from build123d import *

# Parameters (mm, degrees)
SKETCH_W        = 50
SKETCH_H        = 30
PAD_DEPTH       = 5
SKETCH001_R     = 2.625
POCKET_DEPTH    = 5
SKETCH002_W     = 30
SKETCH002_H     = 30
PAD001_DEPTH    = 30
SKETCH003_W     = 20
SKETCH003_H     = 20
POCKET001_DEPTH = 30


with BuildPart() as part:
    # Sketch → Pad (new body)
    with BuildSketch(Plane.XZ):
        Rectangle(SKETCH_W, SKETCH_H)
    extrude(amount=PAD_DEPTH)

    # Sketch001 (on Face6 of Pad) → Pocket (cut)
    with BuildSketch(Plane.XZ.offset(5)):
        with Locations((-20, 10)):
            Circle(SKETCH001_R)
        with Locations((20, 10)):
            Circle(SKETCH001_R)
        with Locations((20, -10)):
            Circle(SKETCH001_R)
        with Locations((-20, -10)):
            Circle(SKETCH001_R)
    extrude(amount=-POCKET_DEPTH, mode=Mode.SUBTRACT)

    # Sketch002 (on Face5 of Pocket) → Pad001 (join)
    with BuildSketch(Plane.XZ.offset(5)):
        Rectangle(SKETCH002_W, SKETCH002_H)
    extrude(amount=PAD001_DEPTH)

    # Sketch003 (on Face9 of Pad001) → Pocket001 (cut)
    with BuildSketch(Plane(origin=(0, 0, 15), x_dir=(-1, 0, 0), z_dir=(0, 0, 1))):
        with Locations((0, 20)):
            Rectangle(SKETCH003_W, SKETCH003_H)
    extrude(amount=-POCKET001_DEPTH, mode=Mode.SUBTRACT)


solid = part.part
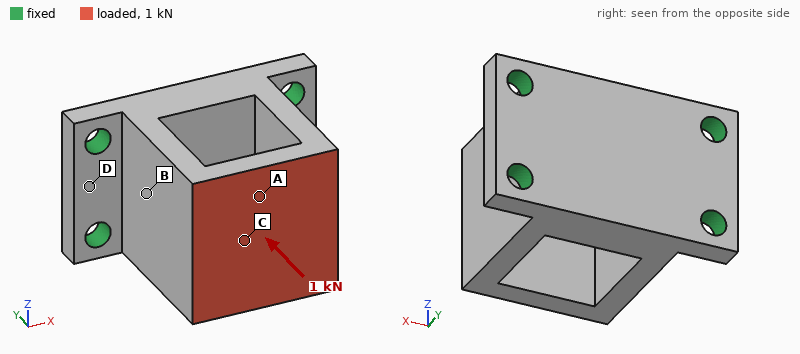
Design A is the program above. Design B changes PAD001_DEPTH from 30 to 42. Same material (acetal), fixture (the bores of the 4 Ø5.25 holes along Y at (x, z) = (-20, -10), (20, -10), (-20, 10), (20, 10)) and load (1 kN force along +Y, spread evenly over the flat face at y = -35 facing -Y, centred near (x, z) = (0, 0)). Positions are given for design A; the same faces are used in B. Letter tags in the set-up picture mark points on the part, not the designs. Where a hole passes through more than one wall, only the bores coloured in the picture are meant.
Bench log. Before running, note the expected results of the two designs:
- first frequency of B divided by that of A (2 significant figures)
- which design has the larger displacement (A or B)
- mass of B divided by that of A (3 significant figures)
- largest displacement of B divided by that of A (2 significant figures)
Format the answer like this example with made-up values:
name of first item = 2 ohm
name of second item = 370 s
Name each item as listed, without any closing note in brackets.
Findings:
first frequency of B divided by that of A = 0.64
which design has the larger displacement = A
mass of B divided by that of A = 1.49
largest displacement of B divided by that of A = 0.52
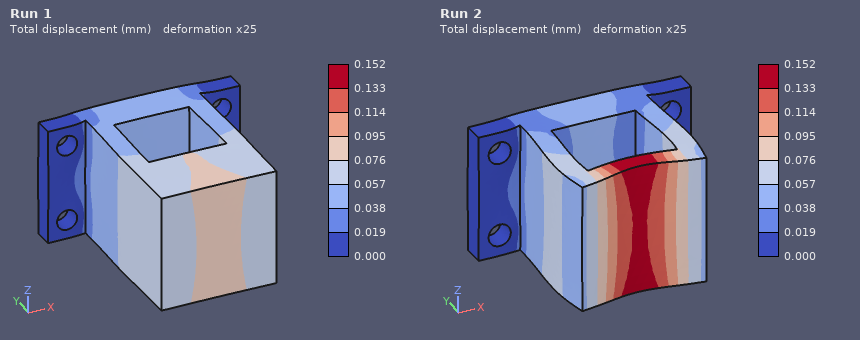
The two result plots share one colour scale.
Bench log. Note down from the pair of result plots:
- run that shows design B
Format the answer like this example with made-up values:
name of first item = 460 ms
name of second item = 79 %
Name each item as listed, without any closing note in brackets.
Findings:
run that shows design B = Run 1
